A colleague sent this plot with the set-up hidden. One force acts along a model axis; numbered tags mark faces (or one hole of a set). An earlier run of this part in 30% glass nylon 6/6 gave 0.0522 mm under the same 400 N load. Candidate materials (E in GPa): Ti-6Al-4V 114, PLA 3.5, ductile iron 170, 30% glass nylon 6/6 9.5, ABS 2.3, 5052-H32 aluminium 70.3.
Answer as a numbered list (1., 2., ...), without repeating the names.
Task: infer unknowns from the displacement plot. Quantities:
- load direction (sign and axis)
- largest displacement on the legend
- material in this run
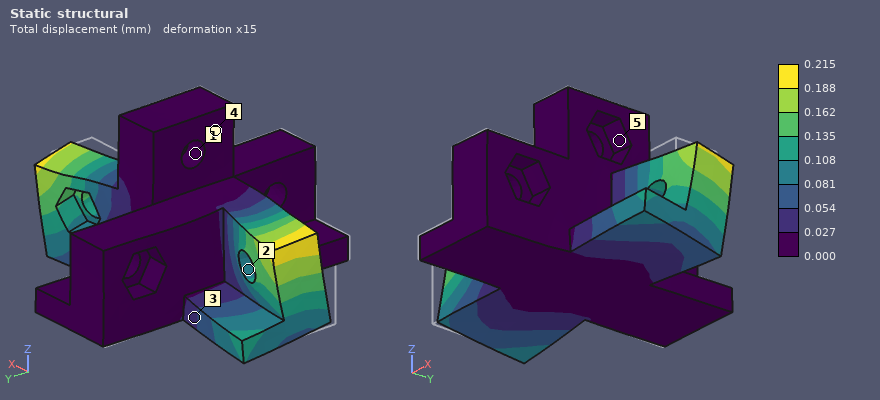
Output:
1. +Y
2. 0.215 mm
3. ABS
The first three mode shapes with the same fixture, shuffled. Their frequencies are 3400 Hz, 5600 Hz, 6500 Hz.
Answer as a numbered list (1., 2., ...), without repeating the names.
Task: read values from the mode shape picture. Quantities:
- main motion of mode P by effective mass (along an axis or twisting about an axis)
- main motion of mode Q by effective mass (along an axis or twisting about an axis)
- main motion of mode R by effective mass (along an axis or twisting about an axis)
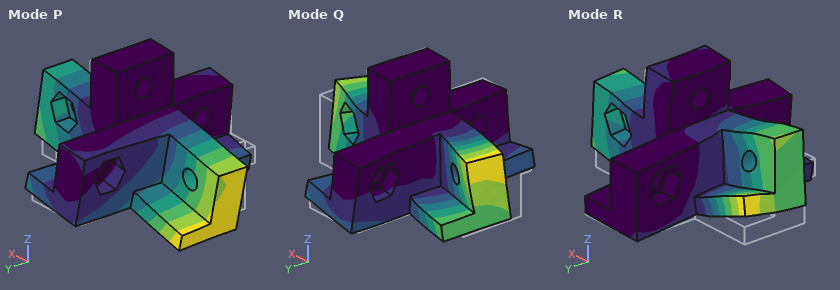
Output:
1. along X
2. twisting about Z
3. along Z
